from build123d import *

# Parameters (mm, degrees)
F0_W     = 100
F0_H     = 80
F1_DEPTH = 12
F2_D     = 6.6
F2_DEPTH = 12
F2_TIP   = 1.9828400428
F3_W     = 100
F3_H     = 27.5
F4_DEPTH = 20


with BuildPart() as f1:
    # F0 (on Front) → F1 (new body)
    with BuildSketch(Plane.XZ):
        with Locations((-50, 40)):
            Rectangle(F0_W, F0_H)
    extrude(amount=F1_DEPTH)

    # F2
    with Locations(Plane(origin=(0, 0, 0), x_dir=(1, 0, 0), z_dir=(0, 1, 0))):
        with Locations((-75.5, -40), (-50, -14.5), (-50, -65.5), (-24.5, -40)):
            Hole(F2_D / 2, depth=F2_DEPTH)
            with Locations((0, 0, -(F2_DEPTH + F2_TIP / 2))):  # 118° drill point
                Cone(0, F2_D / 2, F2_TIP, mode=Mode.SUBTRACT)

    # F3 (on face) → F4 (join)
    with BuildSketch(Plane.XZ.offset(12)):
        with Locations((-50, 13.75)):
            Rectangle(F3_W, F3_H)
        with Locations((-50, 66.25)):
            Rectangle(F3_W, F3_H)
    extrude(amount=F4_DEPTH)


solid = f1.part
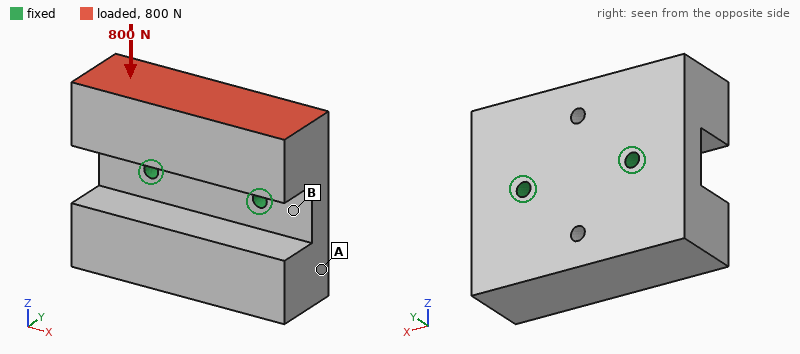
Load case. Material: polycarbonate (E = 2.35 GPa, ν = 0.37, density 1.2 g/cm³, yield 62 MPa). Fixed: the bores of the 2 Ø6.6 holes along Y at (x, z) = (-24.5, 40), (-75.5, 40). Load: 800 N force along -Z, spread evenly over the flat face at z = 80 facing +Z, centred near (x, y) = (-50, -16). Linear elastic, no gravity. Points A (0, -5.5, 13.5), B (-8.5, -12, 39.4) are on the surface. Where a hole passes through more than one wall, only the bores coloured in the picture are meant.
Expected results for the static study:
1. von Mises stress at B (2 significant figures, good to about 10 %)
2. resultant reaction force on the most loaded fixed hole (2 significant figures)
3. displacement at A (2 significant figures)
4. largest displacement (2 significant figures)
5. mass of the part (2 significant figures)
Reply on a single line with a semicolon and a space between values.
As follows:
1.7 MPa; 400 N; 0.039 mm; 0.22 mm; 250 g
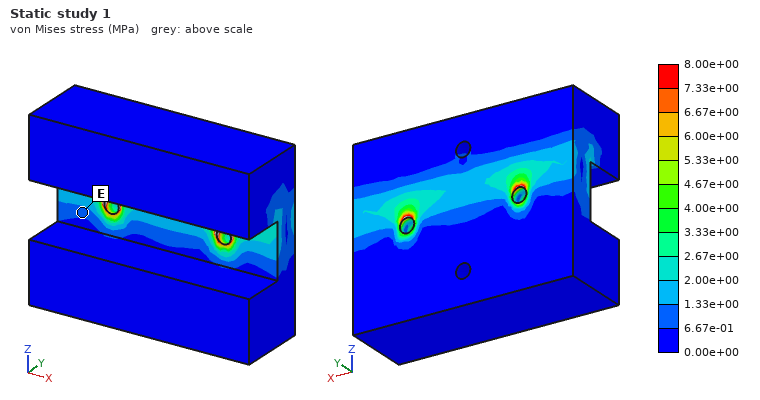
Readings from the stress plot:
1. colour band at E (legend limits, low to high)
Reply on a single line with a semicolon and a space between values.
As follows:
6.67e-01 to 1.33e+00 MPa
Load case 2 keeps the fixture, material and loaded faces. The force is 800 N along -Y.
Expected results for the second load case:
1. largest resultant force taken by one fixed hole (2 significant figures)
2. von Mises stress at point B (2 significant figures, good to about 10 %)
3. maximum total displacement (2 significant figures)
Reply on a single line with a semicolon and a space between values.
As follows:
400 N; 4.8 MPa; 0.76 mm
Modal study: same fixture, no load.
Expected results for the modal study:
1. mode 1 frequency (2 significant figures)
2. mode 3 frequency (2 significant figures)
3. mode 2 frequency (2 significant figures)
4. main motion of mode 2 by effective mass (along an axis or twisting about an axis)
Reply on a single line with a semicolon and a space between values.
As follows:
640 Hz; 1500 Hz; 930 Hz; along Y
